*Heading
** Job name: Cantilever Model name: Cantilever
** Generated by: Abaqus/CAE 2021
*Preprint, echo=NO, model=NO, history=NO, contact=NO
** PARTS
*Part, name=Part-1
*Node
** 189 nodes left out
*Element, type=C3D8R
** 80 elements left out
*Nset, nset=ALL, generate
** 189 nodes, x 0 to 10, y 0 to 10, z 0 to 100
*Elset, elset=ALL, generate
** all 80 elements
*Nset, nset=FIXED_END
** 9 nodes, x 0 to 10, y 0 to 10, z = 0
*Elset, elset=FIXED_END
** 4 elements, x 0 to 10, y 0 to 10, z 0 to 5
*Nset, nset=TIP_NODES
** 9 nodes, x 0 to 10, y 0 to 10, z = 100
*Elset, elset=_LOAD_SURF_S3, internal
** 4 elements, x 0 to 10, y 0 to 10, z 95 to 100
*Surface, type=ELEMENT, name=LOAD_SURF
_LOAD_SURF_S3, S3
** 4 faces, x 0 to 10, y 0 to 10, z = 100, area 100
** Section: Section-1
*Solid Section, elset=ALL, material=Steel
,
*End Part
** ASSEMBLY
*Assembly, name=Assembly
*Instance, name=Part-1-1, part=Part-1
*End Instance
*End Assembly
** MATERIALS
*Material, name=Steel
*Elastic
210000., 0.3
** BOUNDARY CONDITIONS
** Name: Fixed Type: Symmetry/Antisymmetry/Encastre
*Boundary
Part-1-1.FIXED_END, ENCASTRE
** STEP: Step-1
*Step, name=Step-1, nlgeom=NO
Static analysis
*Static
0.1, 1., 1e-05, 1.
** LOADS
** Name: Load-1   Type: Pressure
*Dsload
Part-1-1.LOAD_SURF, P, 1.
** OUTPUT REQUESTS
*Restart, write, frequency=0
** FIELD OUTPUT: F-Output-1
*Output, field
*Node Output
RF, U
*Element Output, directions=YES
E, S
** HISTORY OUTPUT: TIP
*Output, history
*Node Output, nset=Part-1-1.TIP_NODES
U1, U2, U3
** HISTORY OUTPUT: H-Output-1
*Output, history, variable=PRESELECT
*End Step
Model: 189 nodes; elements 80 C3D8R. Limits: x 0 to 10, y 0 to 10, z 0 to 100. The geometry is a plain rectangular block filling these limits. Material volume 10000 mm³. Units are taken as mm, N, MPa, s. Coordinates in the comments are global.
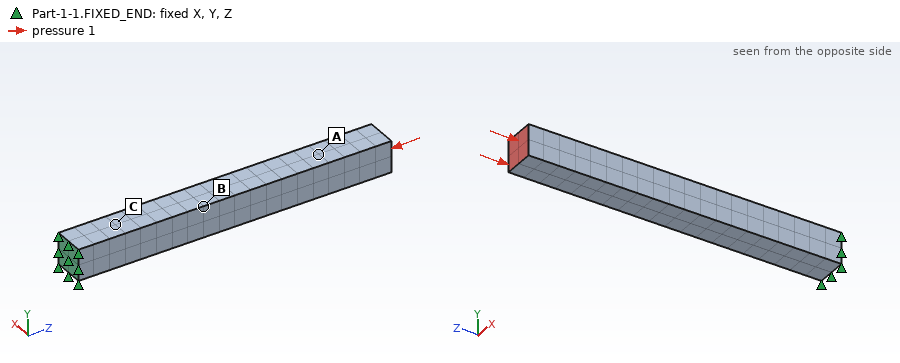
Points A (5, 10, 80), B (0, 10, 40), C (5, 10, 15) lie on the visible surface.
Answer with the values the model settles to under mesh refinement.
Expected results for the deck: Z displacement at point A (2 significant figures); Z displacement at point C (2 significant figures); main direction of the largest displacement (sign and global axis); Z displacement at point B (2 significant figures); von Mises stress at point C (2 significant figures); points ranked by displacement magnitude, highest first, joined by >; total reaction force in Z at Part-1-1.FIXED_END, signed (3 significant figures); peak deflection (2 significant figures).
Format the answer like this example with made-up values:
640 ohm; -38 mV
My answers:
-3.8e-04 mm; -7.0e-05 mm; -Z; -1.9e-04 mm; 1.0 MPa; A > B > C; 100 N; 4.7e-04 mm
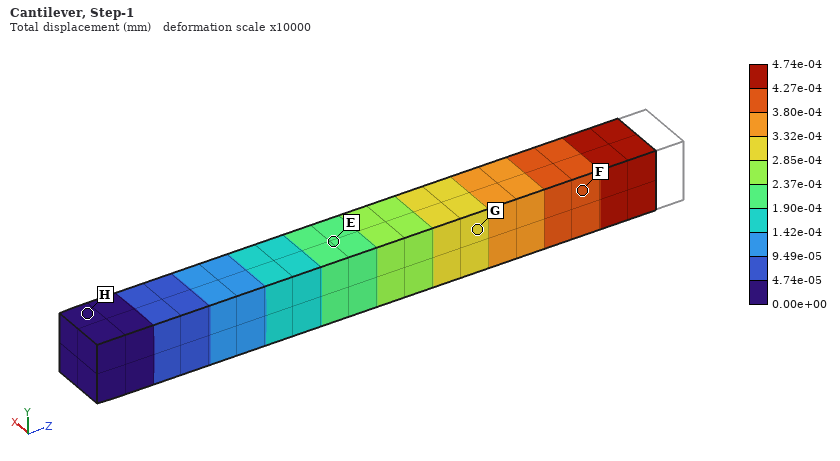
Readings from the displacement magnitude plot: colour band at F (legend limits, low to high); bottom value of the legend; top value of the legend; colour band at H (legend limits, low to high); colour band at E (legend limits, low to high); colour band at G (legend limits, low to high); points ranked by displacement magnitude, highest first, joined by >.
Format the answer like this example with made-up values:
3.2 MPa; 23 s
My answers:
3.80e-04 to 4.27e-04 mm; 0.00e+00 mm; 4.74e-04 mm; 0.00e+00 to 4.74e-05 mm; 1.90e-04 to 2.37e-04 mm; 2.85e-04 to 3.32e-04 mm; F > G > E > H
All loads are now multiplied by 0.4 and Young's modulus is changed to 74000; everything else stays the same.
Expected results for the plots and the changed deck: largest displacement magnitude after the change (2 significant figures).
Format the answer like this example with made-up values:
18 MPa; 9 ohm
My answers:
5.4e-04 mm
